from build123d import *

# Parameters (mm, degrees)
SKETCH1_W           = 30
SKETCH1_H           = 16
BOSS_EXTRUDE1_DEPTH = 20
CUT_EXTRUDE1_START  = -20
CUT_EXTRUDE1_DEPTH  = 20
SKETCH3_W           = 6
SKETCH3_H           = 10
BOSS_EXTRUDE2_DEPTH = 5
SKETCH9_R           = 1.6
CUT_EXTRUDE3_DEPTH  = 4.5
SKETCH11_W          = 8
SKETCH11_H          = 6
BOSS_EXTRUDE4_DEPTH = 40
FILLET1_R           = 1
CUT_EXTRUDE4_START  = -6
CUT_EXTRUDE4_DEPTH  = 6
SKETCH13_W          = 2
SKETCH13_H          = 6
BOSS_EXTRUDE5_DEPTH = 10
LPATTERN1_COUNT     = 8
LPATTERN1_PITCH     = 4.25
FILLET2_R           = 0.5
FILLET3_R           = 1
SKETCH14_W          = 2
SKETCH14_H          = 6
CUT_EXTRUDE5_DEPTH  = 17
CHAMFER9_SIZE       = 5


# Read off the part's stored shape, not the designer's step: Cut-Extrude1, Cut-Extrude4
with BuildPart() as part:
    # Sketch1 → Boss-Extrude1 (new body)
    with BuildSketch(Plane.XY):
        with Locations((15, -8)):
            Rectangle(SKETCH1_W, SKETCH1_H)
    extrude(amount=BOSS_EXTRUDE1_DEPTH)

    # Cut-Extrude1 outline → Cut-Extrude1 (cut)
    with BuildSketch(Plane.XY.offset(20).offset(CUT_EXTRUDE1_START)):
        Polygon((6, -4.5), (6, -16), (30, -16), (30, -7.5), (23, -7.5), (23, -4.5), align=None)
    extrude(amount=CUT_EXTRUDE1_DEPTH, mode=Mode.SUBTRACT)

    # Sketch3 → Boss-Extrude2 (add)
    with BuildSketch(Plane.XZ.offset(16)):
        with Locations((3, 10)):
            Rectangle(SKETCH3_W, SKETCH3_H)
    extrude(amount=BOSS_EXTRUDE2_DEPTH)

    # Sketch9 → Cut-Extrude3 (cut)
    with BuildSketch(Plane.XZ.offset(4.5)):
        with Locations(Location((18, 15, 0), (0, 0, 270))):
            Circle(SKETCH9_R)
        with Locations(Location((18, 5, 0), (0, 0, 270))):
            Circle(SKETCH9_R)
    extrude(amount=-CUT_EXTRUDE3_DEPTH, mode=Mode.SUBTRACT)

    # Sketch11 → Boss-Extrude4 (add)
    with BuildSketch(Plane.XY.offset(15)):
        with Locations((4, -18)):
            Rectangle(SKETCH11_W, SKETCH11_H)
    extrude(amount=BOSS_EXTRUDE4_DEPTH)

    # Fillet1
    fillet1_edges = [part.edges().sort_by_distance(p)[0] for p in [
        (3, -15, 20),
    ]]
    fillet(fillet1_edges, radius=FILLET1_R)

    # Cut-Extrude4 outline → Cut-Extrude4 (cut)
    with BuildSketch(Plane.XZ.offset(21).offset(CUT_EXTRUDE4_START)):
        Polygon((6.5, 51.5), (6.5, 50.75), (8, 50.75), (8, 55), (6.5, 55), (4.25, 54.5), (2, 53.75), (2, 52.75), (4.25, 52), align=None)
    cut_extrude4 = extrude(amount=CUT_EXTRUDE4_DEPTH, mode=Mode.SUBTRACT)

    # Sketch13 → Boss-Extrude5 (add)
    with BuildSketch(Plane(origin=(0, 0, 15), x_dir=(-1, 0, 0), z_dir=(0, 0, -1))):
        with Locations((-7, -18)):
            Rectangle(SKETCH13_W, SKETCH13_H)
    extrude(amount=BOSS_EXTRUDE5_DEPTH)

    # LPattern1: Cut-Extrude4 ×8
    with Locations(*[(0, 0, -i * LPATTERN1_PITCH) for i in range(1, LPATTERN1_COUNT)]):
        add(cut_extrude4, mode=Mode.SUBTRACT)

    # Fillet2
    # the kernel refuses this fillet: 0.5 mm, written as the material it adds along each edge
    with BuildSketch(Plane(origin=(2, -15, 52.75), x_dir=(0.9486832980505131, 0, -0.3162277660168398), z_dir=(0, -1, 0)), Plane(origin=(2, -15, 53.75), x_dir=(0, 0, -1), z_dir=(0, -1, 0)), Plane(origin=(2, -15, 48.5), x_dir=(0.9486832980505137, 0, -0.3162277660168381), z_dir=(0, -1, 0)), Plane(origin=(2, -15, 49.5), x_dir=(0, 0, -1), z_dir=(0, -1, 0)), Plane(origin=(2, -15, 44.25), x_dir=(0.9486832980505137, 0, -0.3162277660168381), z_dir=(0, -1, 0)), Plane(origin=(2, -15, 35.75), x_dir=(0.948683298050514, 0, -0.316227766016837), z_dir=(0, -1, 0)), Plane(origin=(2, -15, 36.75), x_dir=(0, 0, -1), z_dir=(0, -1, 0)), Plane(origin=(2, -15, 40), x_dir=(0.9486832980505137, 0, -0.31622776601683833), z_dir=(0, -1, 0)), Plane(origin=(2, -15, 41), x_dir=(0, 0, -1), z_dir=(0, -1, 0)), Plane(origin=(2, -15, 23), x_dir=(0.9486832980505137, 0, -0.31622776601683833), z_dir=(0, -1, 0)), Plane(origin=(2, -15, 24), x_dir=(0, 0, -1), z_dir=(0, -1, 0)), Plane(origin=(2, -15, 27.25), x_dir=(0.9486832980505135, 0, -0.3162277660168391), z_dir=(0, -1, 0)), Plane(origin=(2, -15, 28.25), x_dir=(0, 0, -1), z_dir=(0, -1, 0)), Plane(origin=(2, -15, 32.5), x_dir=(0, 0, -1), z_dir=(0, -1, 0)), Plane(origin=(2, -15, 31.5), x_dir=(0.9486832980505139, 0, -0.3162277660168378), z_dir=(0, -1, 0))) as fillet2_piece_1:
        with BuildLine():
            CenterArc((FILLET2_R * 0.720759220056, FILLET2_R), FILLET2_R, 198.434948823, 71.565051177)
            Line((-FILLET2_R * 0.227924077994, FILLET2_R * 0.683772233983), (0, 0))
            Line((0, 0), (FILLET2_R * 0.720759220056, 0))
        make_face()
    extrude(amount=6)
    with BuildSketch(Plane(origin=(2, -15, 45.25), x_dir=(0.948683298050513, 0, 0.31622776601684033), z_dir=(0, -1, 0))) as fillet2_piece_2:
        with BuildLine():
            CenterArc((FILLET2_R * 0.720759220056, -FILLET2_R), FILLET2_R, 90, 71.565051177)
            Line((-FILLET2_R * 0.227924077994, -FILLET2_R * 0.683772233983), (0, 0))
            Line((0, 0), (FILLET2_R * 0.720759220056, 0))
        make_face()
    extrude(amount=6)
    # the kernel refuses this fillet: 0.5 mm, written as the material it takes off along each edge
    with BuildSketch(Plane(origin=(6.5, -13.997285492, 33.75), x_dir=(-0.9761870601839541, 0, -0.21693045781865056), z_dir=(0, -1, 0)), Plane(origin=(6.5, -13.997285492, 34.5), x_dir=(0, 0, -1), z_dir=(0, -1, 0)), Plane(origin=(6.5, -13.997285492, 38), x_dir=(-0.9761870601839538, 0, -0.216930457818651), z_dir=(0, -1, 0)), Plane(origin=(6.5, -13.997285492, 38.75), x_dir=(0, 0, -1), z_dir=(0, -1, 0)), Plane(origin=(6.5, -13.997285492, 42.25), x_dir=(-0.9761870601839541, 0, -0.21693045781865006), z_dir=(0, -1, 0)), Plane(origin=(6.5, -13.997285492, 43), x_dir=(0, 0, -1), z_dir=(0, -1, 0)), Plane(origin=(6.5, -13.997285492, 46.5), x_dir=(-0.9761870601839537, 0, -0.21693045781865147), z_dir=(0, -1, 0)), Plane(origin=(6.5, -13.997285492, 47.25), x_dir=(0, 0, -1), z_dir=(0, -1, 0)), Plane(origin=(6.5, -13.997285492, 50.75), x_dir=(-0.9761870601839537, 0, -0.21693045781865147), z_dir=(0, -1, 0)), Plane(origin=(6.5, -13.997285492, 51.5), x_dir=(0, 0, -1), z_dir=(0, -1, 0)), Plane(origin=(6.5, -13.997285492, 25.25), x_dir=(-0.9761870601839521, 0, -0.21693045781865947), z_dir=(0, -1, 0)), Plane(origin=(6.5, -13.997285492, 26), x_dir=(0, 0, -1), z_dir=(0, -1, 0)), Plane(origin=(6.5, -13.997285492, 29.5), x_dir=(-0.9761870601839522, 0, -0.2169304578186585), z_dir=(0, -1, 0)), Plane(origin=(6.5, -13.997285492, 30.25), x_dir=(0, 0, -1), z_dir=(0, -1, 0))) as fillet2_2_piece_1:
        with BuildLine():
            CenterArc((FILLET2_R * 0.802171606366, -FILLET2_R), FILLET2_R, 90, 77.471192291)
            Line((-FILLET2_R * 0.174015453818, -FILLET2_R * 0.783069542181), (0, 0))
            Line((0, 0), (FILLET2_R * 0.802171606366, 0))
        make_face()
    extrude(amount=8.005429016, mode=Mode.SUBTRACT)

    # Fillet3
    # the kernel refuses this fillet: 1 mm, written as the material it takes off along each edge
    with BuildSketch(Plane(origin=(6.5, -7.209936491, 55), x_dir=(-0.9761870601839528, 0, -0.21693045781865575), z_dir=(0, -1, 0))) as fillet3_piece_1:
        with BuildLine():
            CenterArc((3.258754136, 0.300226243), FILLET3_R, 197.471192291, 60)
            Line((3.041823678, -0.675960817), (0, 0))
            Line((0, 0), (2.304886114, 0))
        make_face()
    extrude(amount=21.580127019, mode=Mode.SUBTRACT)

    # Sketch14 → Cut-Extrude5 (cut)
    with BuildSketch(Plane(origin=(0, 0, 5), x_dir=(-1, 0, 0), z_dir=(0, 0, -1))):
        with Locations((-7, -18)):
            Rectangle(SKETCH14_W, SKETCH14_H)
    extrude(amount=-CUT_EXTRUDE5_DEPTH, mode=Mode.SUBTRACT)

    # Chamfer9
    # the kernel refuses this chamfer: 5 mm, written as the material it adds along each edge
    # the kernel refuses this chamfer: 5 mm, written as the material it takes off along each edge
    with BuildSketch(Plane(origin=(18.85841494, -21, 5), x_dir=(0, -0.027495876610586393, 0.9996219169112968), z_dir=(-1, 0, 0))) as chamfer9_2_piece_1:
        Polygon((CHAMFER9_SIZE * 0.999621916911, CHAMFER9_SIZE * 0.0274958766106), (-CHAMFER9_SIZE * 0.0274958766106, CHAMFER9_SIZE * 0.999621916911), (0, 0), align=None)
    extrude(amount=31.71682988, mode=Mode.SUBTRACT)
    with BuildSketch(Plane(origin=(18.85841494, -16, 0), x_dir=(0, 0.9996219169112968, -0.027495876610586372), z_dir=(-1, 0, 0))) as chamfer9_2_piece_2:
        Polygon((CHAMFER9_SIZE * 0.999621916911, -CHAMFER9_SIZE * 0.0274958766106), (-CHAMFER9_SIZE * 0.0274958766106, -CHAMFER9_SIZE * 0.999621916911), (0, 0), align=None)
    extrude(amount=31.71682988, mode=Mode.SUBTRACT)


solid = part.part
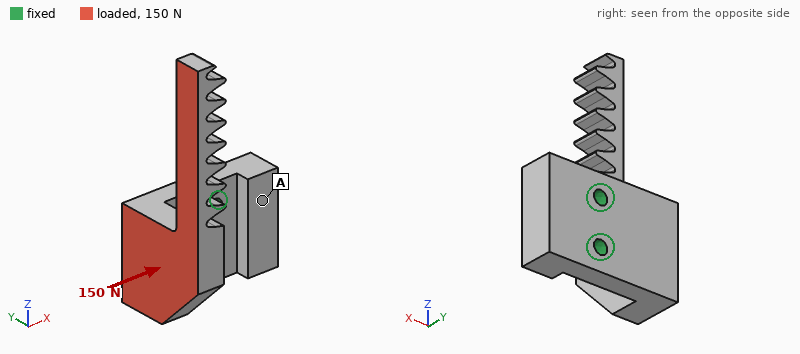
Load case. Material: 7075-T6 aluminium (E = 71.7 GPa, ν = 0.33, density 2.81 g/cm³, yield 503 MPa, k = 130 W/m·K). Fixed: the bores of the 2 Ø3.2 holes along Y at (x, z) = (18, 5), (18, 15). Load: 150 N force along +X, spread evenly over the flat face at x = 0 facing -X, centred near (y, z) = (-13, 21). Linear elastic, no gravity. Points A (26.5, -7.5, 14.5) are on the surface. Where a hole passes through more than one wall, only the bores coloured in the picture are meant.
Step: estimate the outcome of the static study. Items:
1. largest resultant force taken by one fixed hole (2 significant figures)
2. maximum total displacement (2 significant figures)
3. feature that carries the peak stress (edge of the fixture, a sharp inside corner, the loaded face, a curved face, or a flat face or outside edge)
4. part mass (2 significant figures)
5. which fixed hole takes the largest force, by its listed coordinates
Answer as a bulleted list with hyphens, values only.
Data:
- 210 N
- 0.66 mm
- a curved face
- 16 g
- (18, 15)
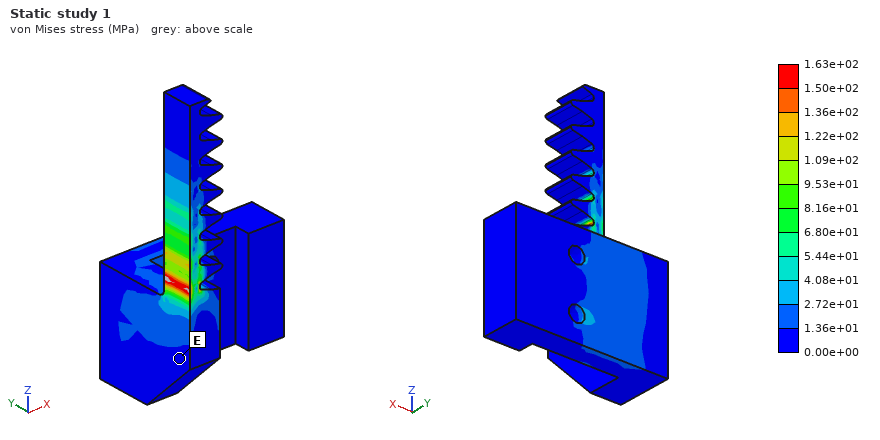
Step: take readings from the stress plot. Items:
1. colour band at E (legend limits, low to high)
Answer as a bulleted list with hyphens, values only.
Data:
- 0.00e+00 to 1.36e+01 MPa
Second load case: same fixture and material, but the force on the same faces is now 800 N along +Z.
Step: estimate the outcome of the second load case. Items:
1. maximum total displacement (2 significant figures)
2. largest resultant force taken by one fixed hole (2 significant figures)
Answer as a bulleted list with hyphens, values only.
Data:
- 0.39 mm
- 1.4 kN
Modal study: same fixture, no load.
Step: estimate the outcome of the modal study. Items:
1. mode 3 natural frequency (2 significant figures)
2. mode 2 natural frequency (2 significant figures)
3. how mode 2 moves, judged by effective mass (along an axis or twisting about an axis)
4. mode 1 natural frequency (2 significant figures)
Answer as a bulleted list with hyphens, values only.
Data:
- 4000 Hz
- 2300 Hz
- along Y
- 1200 Hz
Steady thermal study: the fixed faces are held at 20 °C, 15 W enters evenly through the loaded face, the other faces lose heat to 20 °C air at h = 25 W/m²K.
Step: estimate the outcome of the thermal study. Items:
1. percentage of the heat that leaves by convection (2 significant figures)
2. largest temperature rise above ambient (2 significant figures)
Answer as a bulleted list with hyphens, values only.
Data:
- 10 %
- 65 K
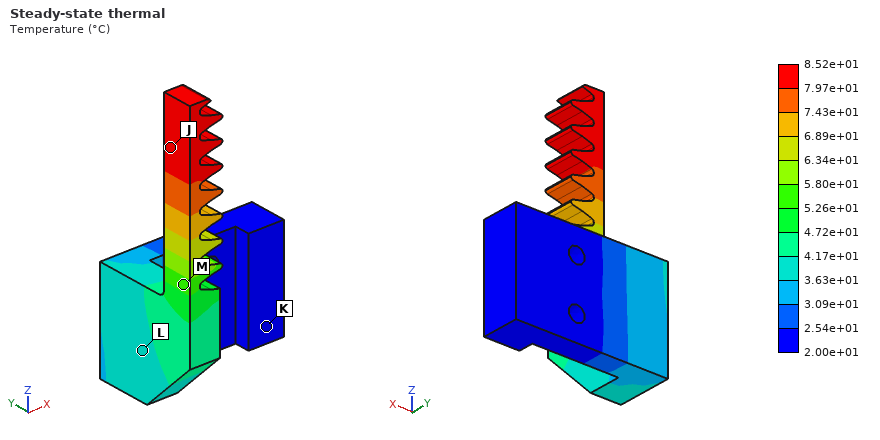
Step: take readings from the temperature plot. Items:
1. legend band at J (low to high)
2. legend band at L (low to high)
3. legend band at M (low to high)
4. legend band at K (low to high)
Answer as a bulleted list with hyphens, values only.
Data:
- 7.97e+01 to 8.52e+01 °C
- 3.63e+01 to 4.17e+01 °C
- 5.26e+01 to 5.80e+01 °C
- 2.00e+01 to 2.54e+01 °C
